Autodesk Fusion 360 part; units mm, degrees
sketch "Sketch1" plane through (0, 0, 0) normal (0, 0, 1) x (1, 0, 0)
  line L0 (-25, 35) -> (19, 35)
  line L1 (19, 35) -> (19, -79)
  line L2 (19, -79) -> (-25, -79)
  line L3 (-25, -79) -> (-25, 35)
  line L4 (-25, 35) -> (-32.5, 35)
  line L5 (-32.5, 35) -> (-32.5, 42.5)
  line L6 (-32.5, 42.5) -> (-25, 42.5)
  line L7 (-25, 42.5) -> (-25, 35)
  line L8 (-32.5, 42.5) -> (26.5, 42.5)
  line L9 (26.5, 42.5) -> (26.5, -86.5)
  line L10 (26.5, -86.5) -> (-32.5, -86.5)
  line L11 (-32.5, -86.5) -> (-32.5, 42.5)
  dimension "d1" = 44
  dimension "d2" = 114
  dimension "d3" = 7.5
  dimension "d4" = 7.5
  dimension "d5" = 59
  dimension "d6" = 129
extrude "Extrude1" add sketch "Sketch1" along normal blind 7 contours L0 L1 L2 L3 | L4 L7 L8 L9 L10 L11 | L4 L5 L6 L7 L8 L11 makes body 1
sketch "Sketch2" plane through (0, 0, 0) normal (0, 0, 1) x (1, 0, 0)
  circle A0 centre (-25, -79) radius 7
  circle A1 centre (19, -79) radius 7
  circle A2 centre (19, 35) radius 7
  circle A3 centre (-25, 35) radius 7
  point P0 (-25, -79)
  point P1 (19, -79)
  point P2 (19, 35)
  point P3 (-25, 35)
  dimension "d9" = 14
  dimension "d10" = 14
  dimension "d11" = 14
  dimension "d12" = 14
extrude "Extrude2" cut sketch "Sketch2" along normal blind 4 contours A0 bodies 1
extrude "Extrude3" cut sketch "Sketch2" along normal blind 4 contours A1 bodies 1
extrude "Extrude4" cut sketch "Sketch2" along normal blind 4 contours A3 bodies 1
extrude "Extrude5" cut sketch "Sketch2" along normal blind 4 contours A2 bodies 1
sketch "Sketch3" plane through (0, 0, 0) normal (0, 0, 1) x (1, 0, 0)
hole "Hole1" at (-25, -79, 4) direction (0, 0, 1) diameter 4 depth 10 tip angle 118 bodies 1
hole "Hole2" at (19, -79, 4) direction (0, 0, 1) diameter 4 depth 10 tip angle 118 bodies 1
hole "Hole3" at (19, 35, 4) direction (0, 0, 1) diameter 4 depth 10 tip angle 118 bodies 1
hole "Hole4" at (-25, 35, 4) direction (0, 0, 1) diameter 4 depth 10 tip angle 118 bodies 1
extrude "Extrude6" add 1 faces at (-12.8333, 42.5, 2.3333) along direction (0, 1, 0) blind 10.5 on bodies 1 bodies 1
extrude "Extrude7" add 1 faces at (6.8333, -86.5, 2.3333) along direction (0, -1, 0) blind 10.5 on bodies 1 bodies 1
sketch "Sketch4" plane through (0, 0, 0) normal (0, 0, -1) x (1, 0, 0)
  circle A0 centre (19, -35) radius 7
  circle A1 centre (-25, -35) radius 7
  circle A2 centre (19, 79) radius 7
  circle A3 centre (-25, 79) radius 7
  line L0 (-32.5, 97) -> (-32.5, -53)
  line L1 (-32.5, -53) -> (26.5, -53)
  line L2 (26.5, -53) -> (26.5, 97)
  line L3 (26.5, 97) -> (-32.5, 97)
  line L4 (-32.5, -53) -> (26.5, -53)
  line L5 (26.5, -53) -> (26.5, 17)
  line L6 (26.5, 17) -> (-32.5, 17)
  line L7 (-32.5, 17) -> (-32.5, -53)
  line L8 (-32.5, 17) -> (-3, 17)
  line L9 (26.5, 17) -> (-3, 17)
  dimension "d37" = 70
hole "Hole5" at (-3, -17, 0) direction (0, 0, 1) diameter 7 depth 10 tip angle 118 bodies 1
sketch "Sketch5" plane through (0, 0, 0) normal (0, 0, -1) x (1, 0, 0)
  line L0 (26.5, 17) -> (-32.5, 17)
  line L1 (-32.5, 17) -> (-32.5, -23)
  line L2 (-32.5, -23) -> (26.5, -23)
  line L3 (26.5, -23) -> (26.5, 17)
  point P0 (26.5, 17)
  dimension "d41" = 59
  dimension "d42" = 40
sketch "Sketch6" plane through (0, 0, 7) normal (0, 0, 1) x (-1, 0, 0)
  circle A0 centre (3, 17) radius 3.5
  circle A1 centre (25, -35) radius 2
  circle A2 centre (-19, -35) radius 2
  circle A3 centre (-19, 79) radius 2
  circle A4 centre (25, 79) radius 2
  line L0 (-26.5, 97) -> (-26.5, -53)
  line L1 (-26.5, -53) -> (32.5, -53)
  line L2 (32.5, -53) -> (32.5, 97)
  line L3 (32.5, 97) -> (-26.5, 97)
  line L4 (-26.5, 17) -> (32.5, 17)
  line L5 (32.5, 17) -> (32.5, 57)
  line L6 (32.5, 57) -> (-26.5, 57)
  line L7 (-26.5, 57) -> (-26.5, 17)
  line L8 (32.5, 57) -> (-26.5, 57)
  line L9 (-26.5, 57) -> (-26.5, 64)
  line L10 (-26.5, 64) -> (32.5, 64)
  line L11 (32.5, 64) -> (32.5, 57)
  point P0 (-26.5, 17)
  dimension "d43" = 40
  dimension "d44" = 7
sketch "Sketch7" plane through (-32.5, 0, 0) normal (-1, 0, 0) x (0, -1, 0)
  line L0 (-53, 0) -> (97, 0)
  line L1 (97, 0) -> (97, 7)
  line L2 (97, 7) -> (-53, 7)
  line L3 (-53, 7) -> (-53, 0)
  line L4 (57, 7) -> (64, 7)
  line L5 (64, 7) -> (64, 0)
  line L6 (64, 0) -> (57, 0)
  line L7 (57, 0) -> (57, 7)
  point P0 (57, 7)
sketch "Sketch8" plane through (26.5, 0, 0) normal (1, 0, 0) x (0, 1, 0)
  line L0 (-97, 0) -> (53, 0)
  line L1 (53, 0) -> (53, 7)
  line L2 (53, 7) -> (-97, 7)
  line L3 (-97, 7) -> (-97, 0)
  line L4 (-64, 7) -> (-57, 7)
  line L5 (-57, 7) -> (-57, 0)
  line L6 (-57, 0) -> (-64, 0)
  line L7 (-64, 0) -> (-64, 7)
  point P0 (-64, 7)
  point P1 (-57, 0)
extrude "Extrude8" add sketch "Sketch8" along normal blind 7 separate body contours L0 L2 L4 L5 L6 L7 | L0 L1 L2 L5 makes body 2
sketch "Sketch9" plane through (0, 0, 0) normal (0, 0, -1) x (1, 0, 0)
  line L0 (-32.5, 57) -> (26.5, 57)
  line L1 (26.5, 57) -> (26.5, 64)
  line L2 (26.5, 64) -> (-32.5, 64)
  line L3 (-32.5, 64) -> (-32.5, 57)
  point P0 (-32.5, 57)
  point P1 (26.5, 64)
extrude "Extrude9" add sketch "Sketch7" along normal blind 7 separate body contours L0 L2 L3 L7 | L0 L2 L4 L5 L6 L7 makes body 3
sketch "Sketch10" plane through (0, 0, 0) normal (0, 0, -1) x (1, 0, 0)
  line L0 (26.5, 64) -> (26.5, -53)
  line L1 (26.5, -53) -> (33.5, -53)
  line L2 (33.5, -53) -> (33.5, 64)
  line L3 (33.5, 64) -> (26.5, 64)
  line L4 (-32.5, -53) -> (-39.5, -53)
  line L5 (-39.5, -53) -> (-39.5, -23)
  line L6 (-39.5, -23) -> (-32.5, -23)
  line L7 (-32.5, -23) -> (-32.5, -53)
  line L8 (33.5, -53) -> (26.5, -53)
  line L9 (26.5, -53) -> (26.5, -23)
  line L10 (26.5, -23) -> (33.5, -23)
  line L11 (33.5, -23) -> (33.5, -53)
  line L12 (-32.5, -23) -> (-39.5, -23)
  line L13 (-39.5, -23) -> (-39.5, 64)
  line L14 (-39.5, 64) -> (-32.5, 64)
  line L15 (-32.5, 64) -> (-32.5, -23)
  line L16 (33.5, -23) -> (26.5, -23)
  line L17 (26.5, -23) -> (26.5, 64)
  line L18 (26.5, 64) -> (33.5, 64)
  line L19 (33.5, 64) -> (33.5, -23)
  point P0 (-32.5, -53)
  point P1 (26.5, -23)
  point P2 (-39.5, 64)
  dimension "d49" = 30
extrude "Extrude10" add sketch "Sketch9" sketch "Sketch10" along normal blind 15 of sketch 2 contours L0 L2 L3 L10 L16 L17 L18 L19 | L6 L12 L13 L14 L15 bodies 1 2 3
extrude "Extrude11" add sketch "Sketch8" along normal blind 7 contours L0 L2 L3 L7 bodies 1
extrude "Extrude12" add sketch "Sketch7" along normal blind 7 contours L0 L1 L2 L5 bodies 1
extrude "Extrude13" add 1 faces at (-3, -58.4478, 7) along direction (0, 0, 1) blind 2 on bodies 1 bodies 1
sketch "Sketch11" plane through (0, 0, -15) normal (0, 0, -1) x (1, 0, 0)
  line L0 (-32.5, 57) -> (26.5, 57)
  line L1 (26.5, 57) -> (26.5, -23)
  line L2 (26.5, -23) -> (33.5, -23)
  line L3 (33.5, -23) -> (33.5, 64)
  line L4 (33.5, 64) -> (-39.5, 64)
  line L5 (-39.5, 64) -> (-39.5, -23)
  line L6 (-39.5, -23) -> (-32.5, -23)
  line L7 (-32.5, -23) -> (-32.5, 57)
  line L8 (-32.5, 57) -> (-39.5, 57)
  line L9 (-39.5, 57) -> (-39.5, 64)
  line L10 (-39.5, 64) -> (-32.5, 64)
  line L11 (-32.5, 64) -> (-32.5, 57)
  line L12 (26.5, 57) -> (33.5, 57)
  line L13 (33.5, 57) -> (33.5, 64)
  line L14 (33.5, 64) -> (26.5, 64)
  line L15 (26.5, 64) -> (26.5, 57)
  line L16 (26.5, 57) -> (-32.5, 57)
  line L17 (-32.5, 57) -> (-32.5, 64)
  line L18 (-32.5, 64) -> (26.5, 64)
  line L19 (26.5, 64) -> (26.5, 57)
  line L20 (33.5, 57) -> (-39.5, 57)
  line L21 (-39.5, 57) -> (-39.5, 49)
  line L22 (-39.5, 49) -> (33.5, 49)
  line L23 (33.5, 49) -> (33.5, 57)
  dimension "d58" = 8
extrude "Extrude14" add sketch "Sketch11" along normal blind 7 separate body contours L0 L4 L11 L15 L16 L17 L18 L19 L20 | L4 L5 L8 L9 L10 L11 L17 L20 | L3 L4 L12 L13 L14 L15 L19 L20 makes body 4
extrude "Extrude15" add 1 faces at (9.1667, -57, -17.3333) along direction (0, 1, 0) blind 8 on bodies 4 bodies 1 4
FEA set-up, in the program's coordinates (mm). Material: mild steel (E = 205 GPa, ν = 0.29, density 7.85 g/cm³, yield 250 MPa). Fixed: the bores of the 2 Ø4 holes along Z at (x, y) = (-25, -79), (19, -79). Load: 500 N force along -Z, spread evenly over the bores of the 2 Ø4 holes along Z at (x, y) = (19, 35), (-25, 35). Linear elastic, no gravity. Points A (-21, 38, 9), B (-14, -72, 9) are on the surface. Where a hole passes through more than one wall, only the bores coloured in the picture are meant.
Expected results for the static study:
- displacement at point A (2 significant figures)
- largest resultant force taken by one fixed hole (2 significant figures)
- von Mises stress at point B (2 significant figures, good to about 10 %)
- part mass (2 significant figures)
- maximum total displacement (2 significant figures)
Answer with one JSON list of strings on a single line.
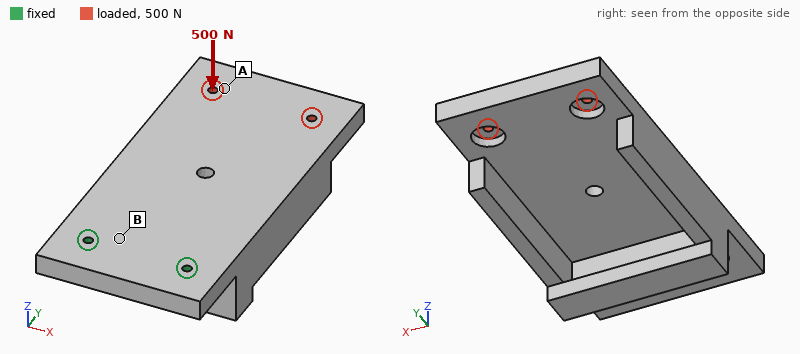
["0.37 mm", "320 N", "56 MPa", "1.0 kg", "0.42 mm"]
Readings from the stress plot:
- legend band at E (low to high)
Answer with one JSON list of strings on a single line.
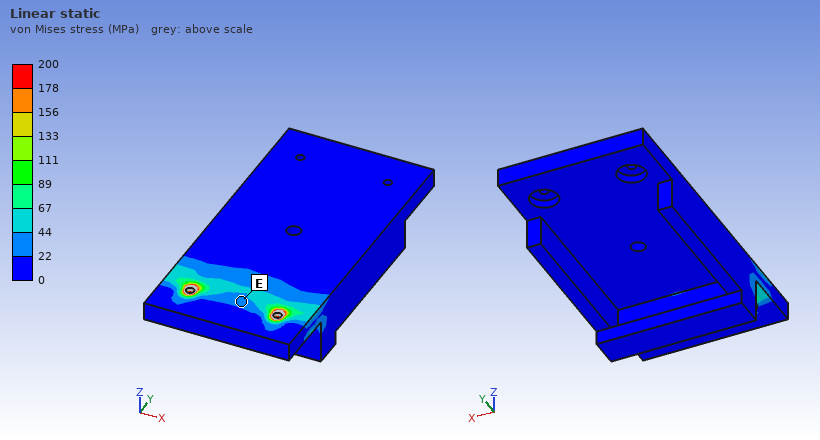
["22 to 44 MPa"]
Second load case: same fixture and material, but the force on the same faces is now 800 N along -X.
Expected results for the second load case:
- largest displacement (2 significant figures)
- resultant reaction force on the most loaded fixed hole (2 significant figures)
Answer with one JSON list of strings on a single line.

["17 µm", "2.1 kN"]
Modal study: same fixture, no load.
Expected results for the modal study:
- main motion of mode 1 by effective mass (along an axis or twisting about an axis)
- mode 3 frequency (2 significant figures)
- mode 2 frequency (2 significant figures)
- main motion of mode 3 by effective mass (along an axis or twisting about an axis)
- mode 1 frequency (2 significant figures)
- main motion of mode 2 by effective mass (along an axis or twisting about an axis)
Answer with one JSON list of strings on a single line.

["along Z", "2100 Hz", "1600 Hz", "along X", "330 Hz", "twisting about Y"]
